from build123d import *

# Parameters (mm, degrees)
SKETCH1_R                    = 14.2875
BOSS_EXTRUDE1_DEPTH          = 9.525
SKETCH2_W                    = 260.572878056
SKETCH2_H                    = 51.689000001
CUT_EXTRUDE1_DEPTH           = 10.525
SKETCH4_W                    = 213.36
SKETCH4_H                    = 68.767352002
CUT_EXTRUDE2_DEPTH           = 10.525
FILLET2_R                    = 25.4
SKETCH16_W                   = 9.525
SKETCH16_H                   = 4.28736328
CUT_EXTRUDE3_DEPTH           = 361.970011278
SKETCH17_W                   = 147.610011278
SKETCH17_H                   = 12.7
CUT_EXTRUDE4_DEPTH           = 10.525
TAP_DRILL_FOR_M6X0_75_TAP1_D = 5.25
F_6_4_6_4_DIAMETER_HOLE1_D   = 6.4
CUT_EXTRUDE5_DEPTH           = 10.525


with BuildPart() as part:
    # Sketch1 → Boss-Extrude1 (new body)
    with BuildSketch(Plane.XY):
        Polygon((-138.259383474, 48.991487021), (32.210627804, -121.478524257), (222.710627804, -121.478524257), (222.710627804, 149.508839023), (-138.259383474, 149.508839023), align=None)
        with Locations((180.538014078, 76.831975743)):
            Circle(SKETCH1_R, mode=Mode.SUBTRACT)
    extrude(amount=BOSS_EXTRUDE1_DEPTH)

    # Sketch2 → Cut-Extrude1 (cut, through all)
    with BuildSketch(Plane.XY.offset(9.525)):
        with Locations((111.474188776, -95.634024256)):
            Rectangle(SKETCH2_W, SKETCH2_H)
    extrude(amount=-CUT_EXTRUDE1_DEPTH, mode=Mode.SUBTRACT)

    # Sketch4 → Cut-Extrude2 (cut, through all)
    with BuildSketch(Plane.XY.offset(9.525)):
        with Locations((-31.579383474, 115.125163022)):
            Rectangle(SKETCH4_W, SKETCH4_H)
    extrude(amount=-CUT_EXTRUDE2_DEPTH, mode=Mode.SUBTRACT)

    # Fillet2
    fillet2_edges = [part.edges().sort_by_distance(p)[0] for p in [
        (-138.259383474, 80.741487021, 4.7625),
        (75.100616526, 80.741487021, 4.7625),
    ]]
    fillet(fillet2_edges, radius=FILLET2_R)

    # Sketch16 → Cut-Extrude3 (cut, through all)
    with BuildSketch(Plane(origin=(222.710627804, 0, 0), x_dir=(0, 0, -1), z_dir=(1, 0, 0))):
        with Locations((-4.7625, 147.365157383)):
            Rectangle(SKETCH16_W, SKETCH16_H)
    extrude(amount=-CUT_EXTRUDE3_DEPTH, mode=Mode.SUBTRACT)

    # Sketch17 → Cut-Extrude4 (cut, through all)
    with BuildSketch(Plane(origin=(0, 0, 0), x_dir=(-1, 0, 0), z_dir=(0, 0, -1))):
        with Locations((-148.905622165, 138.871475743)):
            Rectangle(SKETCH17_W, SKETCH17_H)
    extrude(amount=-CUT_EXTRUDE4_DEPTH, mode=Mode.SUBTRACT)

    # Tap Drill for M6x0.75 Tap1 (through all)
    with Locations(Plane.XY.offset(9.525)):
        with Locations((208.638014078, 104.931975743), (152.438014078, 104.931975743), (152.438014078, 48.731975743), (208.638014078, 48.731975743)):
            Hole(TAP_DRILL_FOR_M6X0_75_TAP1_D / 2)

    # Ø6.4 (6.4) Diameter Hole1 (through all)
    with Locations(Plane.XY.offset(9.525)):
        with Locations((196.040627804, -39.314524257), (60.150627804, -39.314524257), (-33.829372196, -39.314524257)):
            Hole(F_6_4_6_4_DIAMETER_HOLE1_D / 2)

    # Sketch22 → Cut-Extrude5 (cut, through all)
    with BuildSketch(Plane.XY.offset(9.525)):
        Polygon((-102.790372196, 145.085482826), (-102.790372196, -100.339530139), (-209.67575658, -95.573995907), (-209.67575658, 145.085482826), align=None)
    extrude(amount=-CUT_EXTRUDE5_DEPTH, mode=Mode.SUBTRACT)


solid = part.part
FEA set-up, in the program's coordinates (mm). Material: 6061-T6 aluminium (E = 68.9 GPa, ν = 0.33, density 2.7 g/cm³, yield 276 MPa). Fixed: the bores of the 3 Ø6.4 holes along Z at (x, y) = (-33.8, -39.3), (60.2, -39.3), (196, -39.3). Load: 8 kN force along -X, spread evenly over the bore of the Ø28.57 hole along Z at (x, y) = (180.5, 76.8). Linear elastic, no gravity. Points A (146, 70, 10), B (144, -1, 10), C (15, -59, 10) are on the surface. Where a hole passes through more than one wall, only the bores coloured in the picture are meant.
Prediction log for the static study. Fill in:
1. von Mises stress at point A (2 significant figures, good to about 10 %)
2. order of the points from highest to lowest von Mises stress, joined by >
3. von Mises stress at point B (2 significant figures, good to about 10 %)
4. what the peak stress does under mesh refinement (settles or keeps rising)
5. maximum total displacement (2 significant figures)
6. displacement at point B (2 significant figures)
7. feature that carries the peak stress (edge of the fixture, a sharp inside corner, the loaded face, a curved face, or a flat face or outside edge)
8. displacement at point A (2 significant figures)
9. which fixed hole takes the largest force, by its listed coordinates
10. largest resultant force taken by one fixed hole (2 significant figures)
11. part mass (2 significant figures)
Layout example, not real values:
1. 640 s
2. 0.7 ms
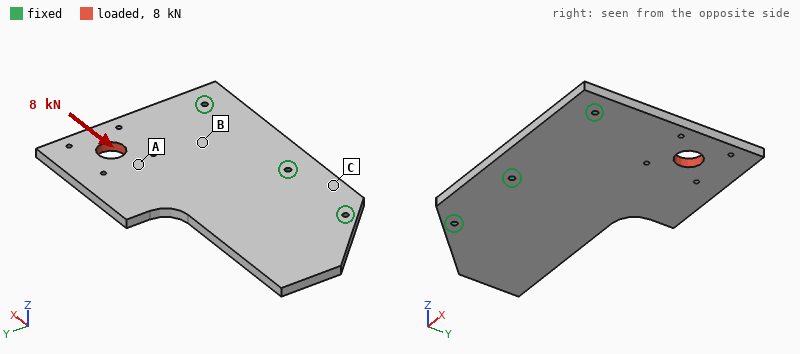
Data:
1. 10 MPa
2. A > B > C
3. 7.1 MPa
4. keeps rising
5. 41 µm
6. 9.5 µm
7. edge of the fixture
8. 27 µm
9. (196, -39.3)
10. 5.3 kN
11. 1.3 kg
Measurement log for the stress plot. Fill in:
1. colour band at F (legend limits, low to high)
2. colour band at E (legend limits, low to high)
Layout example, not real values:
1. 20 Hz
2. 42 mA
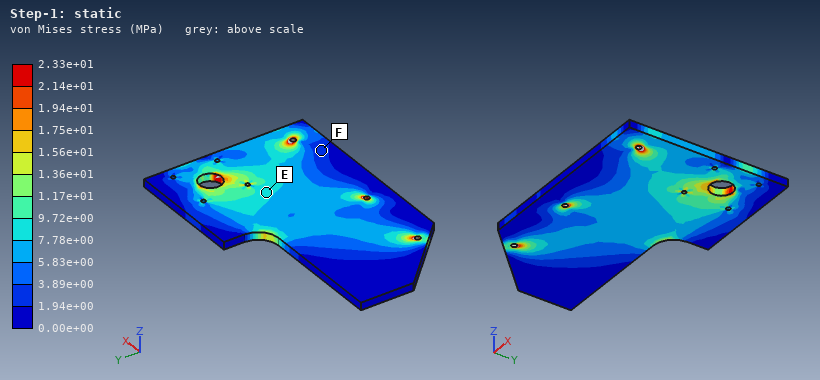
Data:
1. 1.94e+00 to 3.89e+00 MPa
2. 7.78e+00 to 9.72e+00 MPa
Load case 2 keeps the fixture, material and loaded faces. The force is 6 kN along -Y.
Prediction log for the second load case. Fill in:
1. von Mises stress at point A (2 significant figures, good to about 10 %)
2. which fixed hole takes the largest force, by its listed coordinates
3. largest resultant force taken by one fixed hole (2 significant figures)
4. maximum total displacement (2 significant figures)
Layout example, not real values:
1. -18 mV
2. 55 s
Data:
1. 3.8 MPa
2. (196, -39.3)
3. 5.0 kN
4. 21 µm
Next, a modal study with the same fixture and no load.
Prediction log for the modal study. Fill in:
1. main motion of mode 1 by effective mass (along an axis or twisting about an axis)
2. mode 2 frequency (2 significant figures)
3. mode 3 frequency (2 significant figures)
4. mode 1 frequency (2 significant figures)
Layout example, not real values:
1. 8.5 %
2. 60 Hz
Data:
1. along Z
2. 490 Hz
3. 800 Hz
4. 270 Hz
